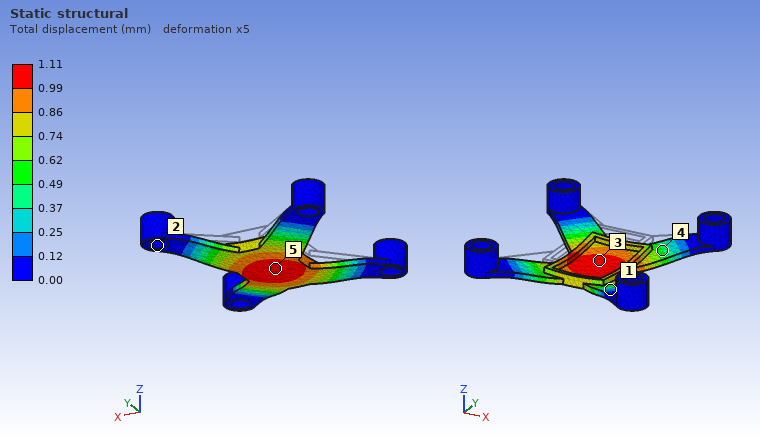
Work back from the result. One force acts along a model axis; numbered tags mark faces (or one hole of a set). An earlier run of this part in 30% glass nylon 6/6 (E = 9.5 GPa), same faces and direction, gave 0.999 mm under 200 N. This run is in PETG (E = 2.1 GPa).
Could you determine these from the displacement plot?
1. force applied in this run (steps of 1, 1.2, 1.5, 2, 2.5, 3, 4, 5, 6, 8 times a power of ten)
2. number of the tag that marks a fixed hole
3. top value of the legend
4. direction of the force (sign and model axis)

50 N
2
1.11 mm
-Z
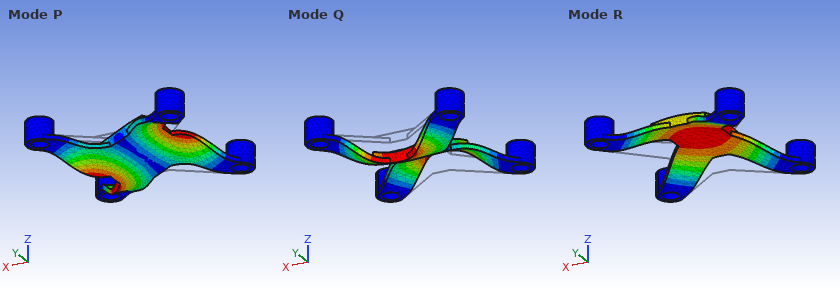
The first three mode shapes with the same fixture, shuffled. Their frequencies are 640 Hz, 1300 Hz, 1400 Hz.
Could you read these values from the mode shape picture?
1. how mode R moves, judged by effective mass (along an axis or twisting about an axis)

along Z
